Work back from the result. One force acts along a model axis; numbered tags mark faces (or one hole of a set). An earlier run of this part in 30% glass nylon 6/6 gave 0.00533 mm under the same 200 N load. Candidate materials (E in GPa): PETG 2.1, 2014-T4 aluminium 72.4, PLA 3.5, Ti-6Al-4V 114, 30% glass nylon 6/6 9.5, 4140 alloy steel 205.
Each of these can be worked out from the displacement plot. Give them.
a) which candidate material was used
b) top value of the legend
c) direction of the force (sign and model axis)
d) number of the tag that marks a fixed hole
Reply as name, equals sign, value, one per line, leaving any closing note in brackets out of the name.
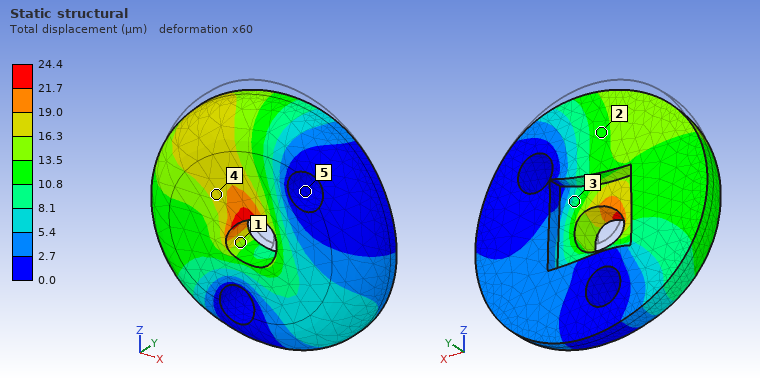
which candidate material was used = PETG
top value of the legend = 24.4 µm
direction of the force = -Z
number of the tag that marks a fixed hole = 5
